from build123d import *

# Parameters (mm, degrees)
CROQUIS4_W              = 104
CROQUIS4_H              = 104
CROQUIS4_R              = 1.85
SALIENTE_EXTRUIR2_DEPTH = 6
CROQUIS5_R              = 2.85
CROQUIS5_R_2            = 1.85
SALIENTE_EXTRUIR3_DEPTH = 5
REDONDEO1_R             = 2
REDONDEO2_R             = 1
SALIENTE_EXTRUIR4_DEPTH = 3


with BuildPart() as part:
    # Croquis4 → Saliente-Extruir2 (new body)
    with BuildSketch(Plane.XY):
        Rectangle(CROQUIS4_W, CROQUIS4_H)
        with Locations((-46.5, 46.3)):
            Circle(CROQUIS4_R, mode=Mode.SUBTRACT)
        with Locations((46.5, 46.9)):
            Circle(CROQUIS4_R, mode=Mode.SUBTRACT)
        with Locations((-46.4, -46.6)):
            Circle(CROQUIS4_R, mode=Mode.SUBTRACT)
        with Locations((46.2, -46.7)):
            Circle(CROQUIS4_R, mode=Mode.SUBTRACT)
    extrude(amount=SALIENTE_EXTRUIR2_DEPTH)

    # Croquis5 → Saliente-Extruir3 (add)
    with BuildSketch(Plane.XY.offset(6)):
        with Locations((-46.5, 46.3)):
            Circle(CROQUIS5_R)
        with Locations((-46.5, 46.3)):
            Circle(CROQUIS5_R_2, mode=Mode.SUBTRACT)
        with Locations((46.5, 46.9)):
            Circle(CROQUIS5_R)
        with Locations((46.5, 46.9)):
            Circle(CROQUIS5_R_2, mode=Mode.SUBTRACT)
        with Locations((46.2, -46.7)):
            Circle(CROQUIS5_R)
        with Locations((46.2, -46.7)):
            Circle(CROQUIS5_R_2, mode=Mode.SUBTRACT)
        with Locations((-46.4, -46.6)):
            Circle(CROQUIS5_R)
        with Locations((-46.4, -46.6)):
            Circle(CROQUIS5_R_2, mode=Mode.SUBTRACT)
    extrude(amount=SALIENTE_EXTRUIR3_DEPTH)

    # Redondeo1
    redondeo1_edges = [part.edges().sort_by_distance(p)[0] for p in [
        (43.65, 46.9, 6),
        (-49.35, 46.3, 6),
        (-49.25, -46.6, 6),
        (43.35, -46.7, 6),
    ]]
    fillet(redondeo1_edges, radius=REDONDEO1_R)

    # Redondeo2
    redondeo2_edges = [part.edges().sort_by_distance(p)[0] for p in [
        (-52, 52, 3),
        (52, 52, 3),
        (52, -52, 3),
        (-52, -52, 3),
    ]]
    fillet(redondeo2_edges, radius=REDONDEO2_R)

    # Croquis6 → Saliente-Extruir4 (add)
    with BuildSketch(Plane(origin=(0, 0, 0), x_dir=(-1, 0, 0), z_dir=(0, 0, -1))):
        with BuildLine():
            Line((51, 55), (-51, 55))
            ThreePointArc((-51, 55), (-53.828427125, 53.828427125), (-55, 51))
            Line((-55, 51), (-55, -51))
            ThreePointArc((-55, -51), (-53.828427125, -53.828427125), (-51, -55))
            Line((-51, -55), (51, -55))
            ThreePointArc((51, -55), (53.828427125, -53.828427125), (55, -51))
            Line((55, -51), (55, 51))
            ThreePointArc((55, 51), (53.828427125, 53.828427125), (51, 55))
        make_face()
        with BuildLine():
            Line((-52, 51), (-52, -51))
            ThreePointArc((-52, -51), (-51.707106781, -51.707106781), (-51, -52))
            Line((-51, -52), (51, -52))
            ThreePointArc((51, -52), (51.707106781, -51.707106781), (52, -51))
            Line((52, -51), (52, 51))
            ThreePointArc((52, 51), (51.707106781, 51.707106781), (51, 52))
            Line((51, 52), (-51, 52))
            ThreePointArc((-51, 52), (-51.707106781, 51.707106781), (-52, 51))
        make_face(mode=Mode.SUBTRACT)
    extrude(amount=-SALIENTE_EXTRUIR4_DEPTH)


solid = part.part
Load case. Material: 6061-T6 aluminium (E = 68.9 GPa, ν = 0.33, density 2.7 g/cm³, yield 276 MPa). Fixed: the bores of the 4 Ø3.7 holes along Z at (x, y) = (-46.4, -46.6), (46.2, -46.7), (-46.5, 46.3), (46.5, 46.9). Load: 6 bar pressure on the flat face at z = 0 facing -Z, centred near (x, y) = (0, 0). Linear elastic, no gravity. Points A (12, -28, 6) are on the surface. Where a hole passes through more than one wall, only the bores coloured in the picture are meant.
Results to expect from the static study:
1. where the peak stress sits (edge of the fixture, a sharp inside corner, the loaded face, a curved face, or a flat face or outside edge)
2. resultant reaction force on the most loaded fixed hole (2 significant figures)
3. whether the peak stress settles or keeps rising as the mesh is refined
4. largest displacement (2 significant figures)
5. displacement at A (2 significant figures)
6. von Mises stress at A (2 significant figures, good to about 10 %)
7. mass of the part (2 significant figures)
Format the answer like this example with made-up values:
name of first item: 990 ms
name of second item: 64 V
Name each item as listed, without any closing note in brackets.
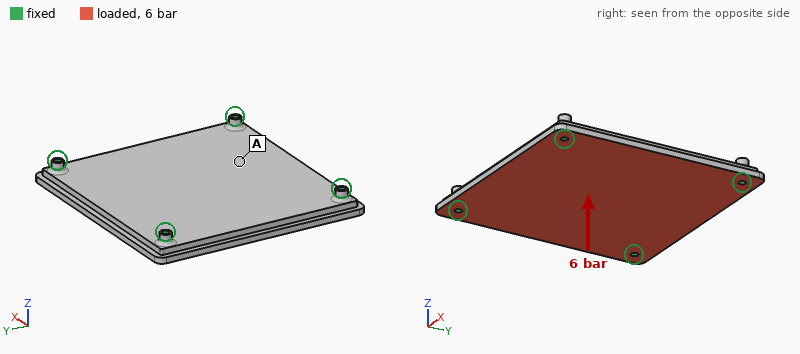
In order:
where the peak stress sits: edge of the fixture
resultant reaction force on the most loaded fixed hole: 1.8 kN
whether the peak stress settles or keeps rising as the mesh is refined: keeps rising
largest displacement: 0.29 mm
displacement at A: 0.21 mm
von Mises stress at A: 41 MPa
mass of the part: 190 g
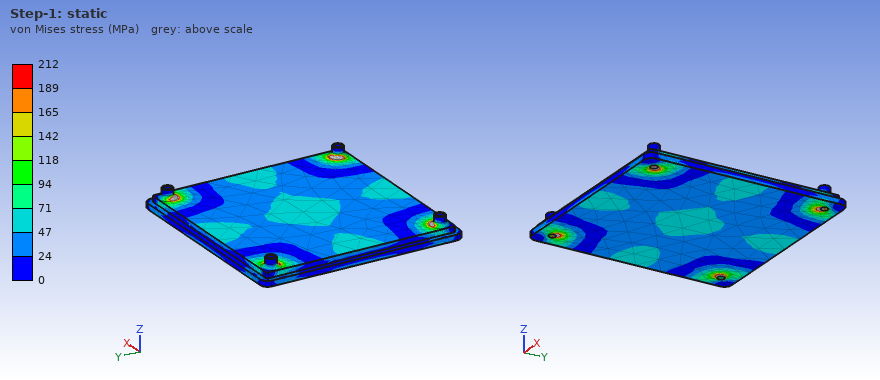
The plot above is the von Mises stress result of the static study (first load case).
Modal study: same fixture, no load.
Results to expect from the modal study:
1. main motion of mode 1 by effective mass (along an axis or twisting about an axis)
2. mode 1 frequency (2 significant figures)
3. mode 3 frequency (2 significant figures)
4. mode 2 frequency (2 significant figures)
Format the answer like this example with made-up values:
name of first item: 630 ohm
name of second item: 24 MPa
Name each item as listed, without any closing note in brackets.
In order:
main motion of mode 1 by effective mass: along Z
mode 1 frequency: 2200 Hz
mode 3 frequency: 3800 Hz
mode 2 frequency: 3700 Hz
